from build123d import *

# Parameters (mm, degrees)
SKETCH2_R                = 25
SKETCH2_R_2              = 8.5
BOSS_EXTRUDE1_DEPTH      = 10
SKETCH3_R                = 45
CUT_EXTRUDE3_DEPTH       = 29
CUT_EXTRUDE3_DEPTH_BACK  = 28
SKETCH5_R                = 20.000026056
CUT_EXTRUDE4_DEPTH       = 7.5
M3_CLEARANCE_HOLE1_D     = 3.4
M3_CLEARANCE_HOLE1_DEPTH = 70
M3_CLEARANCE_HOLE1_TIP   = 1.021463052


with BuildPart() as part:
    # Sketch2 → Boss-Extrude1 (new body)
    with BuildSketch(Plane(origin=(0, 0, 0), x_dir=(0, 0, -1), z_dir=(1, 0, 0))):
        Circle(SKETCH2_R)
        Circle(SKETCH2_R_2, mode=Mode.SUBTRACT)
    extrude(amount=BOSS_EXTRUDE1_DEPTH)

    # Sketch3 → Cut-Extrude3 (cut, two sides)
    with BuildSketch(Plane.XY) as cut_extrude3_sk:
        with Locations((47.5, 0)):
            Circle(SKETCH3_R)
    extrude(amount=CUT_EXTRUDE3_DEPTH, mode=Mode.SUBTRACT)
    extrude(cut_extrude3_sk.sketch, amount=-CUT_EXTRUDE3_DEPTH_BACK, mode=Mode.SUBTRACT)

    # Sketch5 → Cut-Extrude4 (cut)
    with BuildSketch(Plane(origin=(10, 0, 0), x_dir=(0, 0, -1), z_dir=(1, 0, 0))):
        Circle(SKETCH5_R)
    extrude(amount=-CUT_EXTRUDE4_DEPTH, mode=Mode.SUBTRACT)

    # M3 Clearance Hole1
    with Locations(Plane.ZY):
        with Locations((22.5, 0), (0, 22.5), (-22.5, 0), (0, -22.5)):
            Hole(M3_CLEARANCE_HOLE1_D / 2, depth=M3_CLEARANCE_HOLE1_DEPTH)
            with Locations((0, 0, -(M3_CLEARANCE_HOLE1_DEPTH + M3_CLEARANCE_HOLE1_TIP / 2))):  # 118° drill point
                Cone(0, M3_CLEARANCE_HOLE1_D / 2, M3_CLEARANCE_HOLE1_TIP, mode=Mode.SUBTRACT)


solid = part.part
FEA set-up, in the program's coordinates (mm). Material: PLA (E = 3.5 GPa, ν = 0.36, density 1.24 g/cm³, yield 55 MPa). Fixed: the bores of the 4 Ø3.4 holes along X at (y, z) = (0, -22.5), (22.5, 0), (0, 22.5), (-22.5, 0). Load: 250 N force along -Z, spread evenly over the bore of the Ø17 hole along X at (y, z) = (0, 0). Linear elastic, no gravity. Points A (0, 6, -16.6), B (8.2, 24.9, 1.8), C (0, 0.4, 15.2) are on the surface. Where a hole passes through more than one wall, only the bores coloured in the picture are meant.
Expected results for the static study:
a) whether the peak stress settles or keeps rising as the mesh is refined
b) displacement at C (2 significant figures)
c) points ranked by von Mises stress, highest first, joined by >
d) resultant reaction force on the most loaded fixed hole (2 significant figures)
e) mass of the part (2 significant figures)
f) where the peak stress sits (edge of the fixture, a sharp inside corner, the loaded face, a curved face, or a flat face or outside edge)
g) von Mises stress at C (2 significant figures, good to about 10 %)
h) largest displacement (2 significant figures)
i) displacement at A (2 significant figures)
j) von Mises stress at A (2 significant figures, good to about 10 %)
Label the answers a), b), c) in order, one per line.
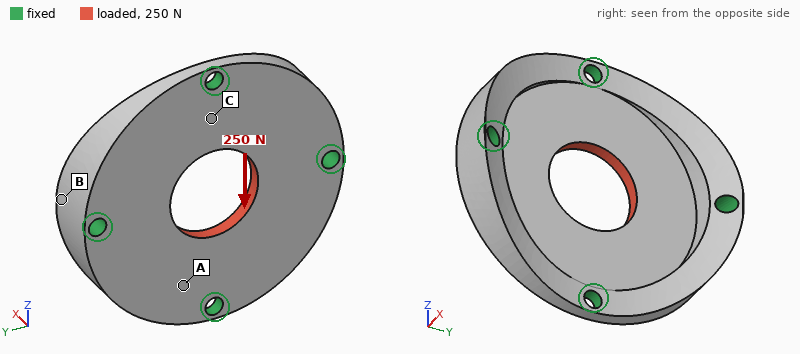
a) keeps rising
b) 6.4 µm
c) C > A > B
d) 69 N
e) 7.8 g
f) edge of the fixture
g) 3.1 MPa
h) 13 µm
i) 7.2 µm
j) 1.7 MPa
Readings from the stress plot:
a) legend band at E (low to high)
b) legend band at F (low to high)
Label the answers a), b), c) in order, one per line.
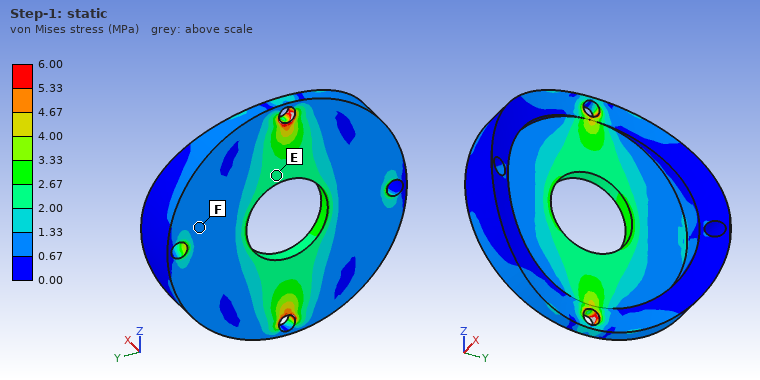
a) 2.00 to 2.67 MPa
b) 0.67 to 1.33 MPa
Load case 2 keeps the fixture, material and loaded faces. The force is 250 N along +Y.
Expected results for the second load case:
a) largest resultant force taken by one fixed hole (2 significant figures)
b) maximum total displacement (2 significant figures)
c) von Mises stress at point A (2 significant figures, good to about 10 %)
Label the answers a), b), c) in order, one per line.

a) 77 N
b) 14 µm
c) 0.76 MPa
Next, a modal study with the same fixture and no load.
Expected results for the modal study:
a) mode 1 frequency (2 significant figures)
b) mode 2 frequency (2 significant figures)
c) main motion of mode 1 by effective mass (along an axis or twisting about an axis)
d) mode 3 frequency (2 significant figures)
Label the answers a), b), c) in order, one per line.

a) 4600 Hz
b) 6000 Hz
c) along X
d) 6100 Hz
